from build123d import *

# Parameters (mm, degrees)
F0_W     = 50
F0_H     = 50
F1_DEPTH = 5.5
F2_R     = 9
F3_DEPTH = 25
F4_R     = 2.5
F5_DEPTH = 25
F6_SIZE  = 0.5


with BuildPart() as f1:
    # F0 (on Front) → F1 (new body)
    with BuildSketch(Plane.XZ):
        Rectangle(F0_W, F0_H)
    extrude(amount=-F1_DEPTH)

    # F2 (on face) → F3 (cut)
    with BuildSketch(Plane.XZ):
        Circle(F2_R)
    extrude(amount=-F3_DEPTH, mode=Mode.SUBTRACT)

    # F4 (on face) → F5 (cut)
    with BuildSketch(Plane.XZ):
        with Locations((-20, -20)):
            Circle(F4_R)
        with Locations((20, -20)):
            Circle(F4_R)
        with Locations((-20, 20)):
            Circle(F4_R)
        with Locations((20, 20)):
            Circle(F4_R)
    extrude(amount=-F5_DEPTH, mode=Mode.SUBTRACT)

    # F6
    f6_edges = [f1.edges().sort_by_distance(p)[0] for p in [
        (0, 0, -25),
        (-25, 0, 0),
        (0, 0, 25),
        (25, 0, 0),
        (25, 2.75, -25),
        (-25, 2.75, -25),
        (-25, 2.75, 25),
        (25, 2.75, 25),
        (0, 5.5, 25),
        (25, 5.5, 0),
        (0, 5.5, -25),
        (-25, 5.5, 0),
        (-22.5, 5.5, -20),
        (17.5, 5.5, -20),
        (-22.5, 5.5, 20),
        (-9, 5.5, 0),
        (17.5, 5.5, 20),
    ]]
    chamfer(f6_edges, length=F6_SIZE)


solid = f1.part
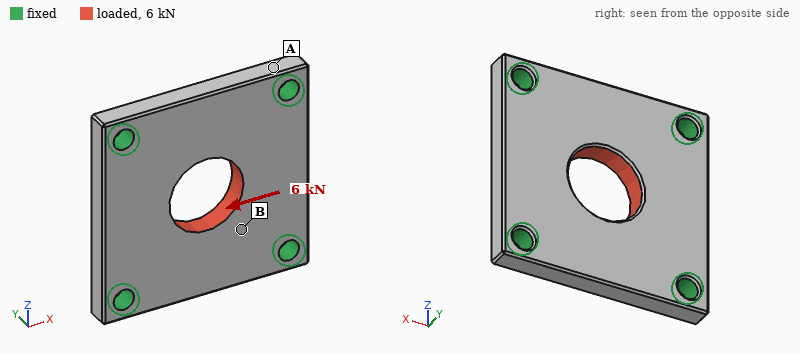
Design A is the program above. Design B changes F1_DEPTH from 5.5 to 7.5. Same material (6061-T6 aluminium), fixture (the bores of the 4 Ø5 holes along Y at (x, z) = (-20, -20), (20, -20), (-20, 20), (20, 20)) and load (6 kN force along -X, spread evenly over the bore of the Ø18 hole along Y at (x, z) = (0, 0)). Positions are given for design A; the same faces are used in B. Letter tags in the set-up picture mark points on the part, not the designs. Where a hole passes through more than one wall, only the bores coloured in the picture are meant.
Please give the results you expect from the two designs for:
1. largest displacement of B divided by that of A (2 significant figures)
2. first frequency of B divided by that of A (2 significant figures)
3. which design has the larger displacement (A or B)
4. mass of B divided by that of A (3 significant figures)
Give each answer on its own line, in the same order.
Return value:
0.73
1.2
A
1.37
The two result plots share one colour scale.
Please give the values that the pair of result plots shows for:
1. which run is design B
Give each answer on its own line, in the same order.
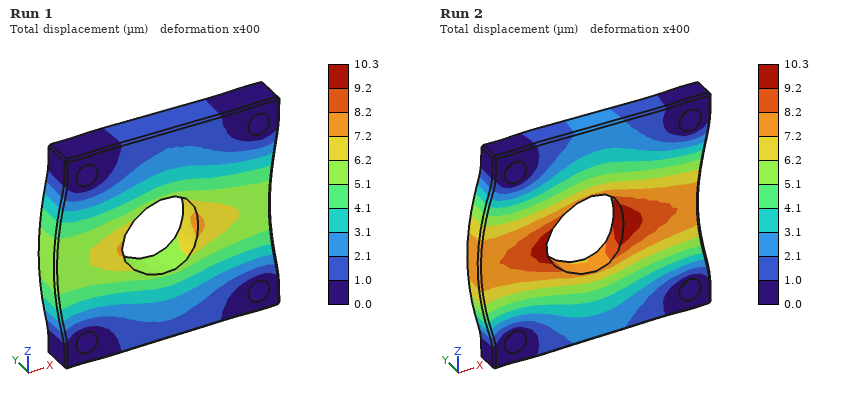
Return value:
Run 1
